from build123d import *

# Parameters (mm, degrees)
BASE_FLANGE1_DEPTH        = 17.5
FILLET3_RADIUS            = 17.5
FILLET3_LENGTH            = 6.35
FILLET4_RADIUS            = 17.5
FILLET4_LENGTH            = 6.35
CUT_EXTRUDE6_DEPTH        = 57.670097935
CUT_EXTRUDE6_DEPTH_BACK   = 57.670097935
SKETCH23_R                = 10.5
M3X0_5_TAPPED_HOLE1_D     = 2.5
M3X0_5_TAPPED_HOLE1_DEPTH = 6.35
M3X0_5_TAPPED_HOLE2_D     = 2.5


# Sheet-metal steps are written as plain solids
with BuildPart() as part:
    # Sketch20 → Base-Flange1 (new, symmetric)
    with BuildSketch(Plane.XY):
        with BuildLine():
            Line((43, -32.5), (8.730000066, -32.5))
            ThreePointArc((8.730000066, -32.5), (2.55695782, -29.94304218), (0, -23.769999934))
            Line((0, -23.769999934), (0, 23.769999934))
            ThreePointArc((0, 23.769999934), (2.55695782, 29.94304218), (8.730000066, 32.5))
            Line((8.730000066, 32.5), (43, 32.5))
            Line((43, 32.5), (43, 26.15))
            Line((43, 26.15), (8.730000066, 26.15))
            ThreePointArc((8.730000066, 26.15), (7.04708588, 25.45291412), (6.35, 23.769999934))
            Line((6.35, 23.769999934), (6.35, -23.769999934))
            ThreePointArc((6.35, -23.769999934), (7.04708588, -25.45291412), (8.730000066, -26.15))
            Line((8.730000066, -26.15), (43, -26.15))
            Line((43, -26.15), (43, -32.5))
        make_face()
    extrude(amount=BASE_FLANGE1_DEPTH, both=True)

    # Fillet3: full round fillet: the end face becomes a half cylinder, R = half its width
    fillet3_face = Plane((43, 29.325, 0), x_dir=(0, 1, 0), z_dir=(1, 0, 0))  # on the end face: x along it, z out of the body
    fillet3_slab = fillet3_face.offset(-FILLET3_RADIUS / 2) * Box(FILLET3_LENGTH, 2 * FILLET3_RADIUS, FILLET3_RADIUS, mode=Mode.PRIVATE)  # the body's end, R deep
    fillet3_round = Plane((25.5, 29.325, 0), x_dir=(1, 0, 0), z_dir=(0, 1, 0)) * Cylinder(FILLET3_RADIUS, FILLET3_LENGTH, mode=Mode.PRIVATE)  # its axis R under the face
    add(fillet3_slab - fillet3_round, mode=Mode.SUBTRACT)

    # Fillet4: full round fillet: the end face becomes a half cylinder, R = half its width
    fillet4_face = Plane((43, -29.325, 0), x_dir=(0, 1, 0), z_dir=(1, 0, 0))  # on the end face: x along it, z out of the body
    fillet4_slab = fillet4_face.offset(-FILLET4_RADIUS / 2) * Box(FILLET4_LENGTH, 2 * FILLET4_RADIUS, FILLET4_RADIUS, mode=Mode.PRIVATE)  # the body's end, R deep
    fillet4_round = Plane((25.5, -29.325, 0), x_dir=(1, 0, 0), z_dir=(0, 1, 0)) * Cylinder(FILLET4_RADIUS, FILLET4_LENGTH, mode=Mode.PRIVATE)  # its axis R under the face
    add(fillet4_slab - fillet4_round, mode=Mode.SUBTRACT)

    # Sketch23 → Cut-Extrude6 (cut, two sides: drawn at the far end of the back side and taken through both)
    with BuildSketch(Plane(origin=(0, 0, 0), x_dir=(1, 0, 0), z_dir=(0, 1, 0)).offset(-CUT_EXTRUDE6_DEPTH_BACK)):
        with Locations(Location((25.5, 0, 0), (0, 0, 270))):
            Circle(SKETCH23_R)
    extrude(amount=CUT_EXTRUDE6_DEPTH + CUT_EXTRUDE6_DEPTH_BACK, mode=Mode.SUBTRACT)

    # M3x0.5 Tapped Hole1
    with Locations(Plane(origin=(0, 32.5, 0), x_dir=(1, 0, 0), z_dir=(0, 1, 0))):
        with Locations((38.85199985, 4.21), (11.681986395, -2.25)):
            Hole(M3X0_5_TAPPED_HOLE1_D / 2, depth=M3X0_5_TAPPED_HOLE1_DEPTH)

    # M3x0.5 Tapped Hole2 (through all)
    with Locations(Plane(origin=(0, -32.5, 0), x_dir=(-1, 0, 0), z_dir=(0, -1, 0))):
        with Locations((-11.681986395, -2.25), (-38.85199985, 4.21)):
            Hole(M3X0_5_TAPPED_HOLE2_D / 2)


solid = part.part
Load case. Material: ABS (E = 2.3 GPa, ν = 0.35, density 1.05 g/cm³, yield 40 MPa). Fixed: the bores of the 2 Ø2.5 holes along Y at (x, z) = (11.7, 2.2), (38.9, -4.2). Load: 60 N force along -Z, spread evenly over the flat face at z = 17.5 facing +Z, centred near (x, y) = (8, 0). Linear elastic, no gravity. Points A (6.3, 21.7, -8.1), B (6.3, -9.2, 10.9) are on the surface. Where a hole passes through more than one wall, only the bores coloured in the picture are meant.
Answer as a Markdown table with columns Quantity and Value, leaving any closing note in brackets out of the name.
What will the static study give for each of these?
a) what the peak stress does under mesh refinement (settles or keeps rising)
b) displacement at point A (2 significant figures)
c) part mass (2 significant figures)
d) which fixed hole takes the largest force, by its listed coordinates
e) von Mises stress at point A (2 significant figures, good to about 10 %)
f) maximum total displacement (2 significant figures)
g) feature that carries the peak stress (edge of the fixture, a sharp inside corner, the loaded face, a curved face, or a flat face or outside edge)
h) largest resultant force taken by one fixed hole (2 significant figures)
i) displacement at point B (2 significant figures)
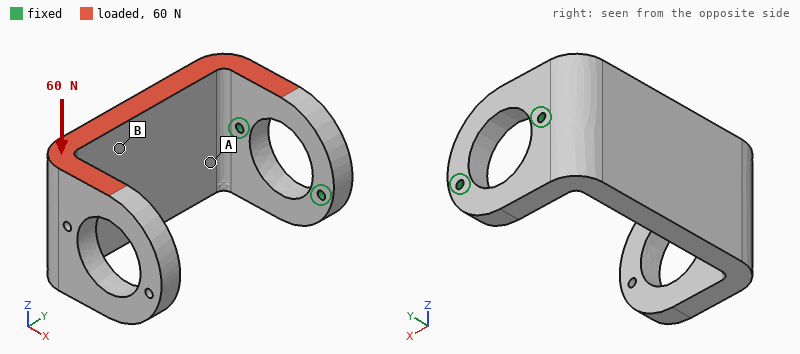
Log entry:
| Quantity | Value |
|---|---|
| what the peak stress does under mesh refinement | keeps rising |
| displacement at point A | 0.15 mm |
| part mass | 25 g |
| which fixed hole takes the largest force, by its listed coordinates | (11.7, 2.2) |
| von Mises stress at point A | 2.6 MPa |
| maximum total displacement | 1.0 mm |
| feature that carries the peak stress | edge of the fixture |
| largest resultant force taken by one fixed hole | 64 N |
| displacement at point B | 0.50 mm |
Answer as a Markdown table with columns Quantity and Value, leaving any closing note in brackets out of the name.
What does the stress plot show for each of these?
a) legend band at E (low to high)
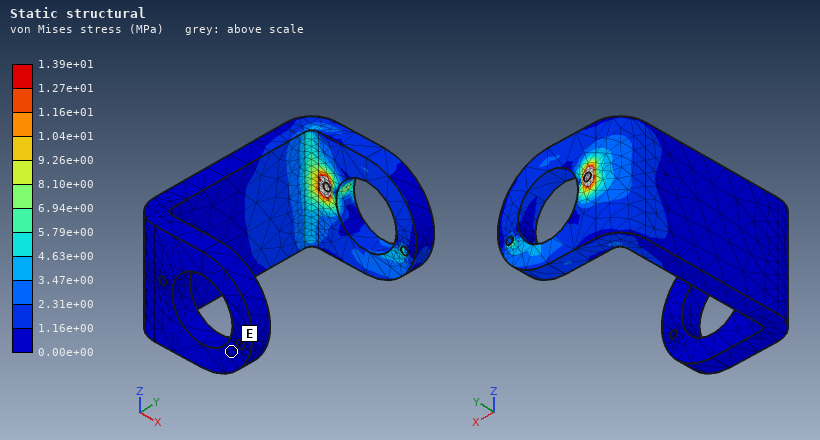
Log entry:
| Quantity | Value |
|---|---|
| legend band at E | 0.00e+00 to 1.16e+00 MPa |
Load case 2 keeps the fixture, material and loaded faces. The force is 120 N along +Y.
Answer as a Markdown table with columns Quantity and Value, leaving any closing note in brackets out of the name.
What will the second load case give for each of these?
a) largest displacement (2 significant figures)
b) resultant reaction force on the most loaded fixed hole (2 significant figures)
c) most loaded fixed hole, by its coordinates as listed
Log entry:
| Quantity | Value |
|---|---|
| largest displacement | 0.99 mm |
| resultant reaction force on the most loaded fixed hole | 130 N |
| most loaded fixed hole, by its coordinates as listed | (11.7, 2.2) |
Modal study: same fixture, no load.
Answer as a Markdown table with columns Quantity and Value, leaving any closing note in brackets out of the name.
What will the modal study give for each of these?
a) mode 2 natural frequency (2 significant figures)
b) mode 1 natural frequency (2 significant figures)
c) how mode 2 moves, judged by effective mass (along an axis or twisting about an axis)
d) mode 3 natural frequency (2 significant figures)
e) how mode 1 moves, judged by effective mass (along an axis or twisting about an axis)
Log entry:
| Quantity | Value |
|---|---|
| mode 2 natural frequency | 290 Hz |
| mode 1 natural frequency | 200 Hz |
| how mode 2 moves, judged by effective mass | along Z |
| mode 3 natural frequency | 680 Hz |
| how mode 1 moves, judged by effective mass | along X |
